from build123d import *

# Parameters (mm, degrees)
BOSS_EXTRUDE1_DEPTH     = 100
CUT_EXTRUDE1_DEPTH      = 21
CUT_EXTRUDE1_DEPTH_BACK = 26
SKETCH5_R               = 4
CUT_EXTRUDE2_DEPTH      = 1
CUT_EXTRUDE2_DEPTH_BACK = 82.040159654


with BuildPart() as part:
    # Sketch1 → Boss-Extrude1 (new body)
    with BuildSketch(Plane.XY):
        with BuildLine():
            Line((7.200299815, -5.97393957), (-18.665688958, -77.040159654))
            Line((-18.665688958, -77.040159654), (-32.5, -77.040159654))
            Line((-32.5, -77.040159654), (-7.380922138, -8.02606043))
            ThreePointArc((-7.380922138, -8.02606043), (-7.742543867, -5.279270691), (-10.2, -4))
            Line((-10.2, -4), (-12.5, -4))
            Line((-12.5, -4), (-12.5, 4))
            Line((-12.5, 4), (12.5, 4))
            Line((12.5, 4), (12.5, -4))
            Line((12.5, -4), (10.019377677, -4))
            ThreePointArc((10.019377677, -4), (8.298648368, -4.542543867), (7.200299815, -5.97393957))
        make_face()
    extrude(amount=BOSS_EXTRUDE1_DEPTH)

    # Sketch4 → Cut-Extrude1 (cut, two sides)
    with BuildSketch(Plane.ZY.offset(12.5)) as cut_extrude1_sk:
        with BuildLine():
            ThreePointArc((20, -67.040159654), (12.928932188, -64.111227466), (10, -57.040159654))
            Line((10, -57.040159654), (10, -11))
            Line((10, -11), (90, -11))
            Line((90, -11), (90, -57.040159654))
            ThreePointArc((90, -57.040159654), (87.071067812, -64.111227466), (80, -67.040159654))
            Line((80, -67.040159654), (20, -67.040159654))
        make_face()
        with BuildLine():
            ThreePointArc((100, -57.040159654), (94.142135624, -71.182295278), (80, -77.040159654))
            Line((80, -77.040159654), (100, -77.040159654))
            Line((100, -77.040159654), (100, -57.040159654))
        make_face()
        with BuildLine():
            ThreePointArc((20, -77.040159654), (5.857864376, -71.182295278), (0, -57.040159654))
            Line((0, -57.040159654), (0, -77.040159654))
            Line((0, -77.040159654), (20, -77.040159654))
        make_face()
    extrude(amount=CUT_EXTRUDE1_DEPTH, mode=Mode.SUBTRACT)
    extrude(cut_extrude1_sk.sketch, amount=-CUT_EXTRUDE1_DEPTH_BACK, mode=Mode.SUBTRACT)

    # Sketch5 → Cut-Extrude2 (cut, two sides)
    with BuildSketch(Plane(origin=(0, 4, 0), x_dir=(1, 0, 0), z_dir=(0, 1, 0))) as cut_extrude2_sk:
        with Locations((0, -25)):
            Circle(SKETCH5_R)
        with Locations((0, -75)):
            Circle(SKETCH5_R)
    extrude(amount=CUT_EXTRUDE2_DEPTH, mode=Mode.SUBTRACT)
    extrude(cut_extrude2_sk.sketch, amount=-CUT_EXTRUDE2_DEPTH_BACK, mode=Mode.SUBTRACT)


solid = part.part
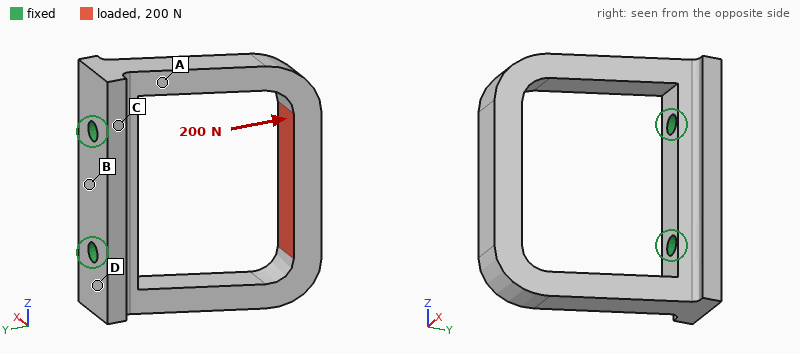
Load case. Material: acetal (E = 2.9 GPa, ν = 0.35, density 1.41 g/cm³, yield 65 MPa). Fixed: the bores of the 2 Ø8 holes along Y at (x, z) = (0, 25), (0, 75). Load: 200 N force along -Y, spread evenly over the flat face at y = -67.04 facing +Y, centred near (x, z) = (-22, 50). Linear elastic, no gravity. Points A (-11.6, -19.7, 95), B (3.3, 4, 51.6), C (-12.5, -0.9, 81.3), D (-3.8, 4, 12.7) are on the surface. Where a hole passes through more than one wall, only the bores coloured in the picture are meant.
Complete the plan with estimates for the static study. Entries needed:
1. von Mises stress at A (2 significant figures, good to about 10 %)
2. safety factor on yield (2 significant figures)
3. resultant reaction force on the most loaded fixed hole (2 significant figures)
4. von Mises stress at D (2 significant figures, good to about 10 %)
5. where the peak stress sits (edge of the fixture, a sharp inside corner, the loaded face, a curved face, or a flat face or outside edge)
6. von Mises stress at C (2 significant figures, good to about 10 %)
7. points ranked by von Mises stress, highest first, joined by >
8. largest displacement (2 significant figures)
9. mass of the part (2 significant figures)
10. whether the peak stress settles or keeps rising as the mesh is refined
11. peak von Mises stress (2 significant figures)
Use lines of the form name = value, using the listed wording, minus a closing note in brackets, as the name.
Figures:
von Mises stress at A = 6.8 MPa
safety factor on yield = 5.6
resultant reaction force on the most loaded fixed hole = 110 N
von Mises stress at D = 3.4 MPa
where the peak stress sits = a curved face
von Mises stress at C = 2.0 MPa
points ranked by von Mises stress, highest first, joined by > = A > D > C > B
largest displacement = 1.3 mm
mass of the part = 79 g
whether the peak stress settles or keeps rising as the mesh is refined = settles
peak von Mises stress = 12 MPa
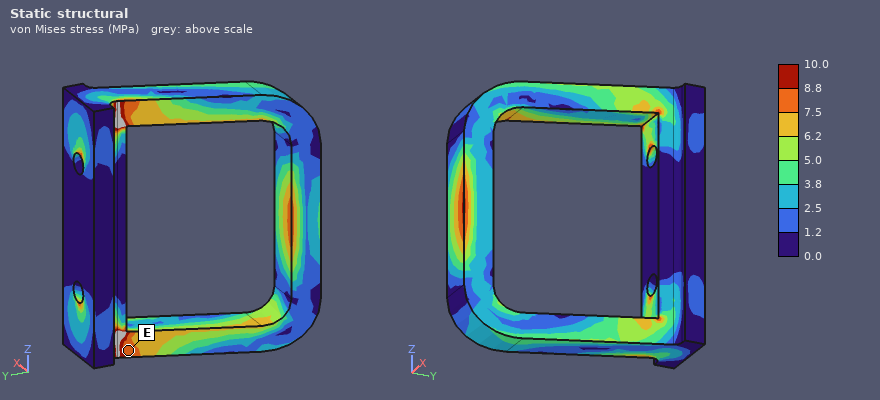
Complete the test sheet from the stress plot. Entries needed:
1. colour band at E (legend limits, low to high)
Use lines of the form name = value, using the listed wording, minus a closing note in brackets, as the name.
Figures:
colour band at E = 7.5 to 8.8 MPa
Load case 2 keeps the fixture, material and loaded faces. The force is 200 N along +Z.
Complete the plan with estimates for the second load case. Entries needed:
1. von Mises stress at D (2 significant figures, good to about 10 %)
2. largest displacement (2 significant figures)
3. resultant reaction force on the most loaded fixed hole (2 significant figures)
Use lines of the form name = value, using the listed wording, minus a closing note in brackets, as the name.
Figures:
von Mises stress at D = 4.9 MPa
largest displacement = 1.4 mm
resultant reaction force on the most loaded fixed hole = 130 N
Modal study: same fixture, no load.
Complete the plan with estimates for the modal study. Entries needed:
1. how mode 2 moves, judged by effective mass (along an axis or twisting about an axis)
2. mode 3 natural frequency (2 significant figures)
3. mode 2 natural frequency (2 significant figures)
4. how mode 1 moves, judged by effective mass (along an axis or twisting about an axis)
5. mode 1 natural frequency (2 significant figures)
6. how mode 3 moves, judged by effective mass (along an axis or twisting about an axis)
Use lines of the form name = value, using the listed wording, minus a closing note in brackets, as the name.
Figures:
how mode 2 moves, judged by effective mass = along Z
mode 3 natural frequency = 560 Hz
mode 2 natural frequency = 400 Hz
how mode 1 moves, judged by effective mass = along X
mode 1 natural frequency = 270 Hz
how mode 3 moves, judged by effective mass = twisting about Y
